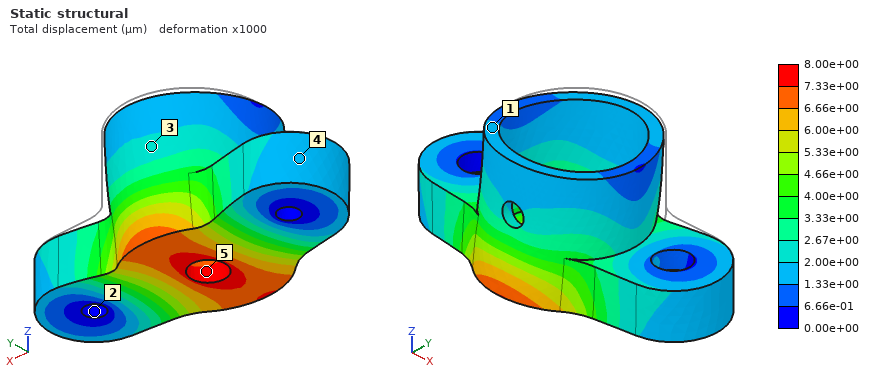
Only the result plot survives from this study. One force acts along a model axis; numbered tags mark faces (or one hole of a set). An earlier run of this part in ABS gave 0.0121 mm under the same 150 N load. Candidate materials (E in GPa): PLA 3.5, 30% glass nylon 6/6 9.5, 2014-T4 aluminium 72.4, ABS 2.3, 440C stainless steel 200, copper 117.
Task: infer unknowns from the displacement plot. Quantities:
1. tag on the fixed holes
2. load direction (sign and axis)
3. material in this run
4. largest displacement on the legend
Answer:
2
-Y
PLA
8.00e+00 µm
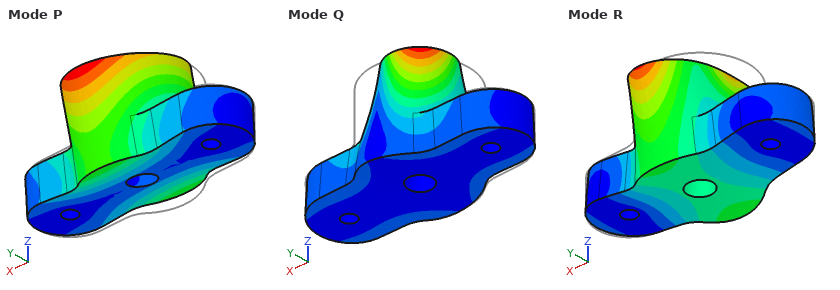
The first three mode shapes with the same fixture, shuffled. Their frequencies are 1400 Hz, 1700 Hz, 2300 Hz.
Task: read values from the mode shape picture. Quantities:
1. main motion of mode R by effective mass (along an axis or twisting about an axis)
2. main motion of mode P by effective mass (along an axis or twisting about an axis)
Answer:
along Z
along Y
